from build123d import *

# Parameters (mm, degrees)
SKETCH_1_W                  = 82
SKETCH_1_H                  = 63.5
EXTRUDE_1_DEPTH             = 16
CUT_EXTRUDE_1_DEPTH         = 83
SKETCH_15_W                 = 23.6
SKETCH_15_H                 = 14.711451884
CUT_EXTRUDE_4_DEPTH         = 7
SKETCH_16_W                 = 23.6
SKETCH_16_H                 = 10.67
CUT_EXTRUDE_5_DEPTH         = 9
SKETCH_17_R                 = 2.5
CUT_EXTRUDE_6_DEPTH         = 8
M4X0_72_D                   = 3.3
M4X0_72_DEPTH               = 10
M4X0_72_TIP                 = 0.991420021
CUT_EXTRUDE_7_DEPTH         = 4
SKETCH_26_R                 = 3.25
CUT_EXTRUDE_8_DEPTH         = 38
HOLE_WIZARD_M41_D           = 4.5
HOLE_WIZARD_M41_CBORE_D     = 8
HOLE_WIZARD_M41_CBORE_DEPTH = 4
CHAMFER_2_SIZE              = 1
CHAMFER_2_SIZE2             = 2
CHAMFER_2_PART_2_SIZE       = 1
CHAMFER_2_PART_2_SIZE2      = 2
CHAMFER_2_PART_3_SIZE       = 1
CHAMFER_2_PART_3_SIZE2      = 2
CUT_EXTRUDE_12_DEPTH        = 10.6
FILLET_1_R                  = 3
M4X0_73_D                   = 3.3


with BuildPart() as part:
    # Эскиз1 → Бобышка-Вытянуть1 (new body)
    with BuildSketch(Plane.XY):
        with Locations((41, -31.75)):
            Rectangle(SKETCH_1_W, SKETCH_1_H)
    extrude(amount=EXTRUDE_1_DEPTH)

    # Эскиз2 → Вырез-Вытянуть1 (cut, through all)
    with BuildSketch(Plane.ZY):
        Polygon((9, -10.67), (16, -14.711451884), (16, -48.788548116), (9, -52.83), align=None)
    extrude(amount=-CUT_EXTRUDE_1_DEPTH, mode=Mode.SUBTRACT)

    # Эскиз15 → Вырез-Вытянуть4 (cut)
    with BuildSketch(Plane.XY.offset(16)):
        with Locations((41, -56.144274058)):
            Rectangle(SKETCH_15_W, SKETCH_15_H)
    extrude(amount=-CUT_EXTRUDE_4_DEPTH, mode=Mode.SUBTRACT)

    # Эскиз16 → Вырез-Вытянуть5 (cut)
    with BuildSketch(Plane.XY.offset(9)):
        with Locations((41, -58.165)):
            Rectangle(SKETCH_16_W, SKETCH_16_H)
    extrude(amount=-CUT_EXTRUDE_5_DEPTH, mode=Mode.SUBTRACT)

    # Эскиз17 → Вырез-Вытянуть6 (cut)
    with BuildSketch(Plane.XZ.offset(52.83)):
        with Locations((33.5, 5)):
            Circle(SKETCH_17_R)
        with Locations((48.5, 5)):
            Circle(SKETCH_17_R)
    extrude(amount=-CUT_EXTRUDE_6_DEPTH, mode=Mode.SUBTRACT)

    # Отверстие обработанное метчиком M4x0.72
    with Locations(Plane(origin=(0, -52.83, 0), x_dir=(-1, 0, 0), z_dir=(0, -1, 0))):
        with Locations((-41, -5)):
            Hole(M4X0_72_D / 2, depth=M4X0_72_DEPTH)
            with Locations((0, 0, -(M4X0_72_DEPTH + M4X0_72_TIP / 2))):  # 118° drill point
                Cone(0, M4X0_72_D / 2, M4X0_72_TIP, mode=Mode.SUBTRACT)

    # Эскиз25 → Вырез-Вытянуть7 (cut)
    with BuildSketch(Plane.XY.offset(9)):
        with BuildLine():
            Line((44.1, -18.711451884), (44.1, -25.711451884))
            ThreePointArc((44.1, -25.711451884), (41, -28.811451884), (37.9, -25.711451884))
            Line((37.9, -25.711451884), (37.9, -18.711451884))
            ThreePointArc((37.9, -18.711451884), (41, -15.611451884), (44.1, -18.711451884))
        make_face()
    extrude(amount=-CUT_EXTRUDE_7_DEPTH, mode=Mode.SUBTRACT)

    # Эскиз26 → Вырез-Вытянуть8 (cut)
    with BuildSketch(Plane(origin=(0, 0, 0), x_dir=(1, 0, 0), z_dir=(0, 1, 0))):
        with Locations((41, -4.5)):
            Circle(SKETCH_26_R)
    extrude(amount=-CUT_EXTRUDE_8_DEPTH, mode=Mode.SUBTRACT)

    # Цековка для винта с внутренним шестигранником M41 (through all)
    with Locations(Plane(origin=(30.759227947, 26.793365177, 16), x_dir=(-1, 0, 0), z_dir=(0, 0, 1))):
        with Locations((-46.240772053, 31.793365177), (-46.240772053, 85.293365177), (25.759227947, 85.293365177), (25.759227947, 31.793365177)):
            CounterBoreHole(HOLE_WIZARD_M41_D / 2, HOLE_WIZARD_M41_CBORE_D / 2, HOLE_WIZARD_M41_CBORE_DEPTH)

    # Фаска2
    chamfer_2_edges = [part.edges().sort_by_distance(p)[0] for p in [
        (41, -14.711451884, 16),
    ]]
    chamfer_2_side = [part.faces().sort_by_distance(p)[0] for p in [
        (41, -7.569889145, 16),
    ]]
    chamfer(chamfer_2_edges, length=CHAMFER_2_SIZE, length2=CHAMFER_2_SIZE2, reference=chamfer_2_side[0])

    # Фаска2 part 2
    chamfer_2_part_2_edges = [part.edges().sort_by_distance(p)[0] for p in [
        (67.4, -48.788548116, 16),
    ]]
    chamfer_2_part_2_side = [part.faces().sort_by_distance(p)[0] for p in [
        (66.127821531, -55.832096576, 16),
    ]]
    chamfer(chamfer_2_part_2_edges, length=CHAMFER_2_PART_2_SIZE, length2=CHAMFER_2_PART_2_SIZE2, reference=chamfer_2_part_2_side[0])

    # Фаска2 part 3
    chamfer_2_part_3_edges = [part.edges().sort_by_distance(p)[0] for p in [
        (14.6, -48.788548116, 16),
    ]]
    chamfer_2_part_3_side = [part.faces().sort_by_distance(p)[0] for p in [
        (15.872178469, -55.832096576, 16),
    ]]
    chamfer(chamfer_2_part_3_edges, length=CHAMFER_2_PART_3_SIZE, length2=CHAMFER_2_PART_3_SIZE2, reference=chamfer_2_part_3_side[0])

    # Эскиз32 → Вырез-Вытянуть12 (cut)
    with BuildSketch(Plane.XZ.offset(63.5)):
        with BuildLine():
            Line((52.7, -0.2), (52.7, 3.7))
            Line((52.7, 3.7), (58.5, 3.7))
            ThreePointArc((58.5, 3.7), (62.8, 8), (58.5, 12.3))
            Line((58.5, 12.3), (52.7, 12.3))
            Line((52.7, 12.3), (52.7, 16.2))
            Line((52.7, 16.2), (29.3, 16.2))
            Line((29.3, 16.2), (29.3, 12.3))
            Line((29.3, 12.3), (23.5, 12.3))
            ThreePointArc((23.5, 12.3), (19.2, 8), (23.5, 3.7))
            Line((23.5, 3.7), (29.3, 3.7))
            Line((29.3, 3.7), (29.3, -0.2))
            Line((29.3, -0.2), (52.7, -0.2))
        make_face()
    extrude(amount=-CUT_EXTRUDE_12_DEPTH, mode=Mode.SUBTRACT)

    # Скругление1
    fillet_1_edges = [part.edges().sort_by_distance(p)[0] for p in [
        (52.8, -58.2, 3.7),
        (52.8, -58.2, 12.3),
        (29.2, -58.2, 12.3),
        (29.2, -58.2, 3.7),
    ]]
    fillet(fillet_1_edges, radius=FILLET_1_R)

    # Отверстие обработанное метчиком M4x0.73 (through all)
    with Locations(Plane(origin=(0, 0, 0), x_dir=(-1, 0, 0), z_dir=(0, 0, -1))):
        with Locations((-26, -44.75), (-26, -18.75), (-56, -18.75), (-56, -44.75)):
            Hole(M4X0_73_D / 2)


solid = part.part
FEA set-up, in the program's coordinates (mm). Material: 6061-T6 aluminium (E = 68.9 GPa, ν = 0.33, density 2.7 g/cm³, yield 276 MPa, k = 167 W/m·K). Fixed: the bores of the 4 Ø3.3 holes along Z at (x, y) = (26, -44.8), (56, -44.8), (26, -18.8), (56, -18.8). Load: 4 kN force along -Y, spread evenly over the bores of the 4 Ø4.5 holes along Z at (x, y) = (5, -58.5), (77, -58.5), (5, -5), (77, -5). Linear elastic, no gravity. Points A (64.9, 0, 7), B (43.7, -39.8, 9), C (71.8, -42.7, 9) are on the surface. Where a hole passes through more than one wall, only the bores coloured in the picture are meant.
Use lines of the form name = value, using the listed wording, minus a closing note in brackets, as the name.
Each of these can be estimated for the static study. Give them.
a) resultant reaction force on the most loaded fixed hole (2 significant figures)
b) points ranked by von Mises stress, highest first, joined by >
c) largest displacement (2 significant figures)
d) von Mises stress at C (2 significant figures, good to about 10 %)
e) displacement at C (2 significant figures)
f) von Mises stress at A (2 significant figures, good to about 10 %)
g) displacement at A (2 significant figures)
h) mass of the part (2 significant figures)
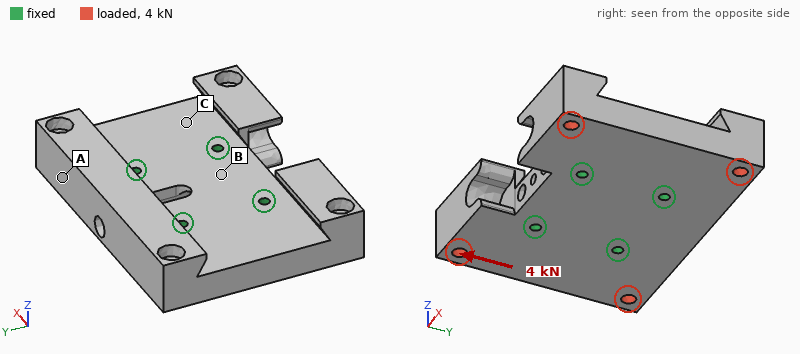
resultant reaction force on the most loaded fixed hole = 1.2 kN
points ranked by von Mises stress, highest first, joined by > = C > A > B
largest displacement = 14 µm
von Mises stress at C = 11 MPa
displacement at C = 5.1 µm
von Mises stress at A = 6.3 MPa
displacement at A = 5.2 µm
mass of the part = 140 g
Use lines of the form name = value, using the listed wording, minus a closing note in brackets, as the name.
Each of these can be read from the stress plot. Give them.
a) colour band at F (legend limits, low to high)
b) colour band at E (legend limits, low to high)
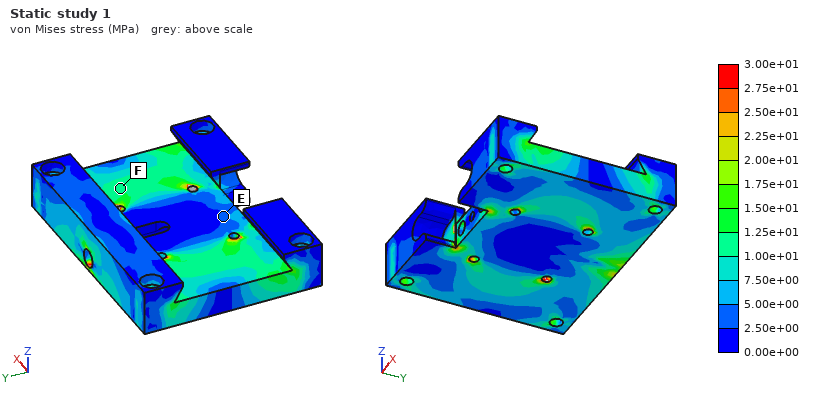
colour band at F = 1.00e+01 to 1.25e+01 MPa
colour band at E = 2.50e+00 to 5.00e+00 MPa
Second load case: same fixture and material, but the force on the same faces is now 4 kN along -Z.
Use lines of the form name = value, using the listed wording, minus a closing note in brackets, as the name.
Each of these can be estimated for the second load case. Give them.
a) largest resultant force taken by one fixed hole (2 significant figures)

largest resultant force taken by one fixed hole = 1.2 kN
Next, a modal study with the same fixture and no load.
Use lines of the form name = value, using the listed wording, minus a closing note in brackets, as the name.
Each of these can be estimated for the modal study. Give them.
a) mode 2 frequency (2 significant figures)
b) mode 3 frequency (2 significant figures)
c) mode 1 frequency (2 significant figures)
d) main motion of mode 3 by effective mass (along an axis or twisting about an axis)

mode 2 frequency = 6900 Hz
mode 3 frequency = 8200 Hz
mode 1 frequency = 6900 Hz
main motion of mode 3 by effective mass = twisting about Y
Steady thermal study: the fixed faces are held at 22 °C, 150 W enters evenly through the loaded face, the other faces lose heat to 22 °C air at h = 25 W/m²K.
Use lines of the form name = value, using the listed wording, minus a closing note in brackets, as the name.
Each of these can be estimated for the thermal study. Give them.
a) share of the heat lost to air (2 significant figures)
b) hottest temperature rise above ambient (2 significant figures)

share of the heat lost to air = 3.8 %
hottest temperature rise above ambient = 32 K
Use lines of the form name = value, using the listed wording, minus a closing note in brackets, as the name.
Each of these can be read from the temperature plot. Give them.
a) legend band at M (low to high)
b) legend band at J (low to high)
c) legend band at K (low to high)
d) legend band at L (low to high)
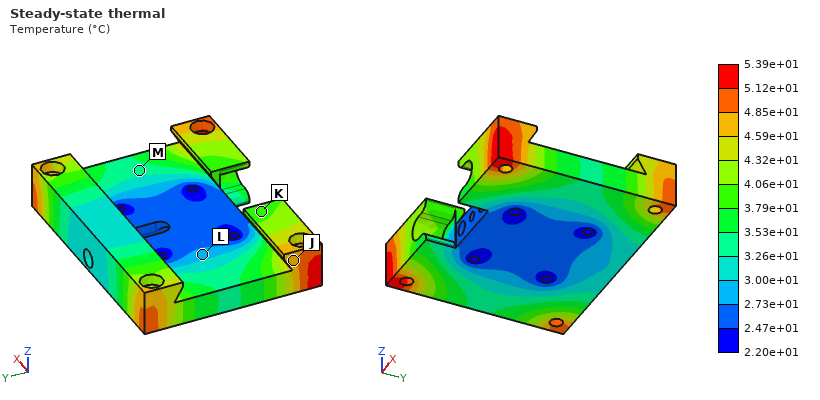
legend band at M = 3.26e+01 to 3.53e+01 °C
legend band at J = 4.59e+01 to 4.85e+01 °C
legend band at K = 3.79e+01 to 4.06e+01 °C
legend band at L = 2.73e+01 to 3.00e+01 °C
